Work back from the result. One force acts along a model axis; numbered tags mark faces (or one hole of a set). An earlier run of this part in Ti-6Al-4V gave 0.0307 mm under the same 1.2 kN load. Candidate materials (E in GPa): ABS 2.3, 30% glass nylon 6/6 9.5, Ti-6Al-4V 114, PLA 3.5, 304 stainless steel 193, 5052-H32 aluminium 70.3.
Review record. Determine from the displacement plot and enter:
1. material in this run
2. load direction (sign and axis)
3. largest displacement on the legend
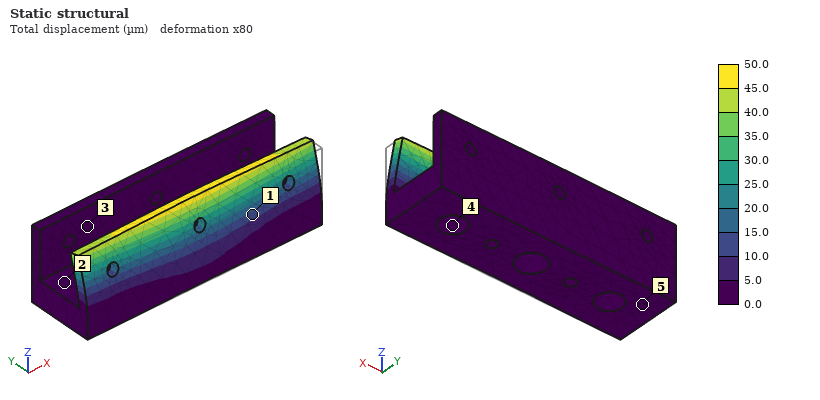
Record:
5052-H32 aluminium
+Y
50.0 µm
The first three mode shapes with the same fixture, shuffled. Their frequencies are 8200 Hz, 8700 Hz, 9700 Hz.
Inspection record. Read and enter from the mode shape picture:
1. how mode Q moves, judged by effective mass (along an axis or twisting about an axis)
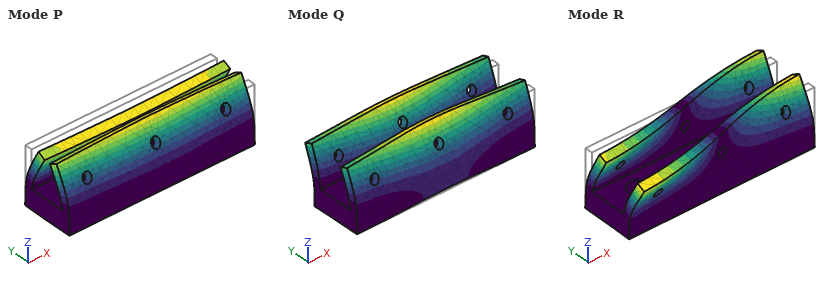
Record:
along Y
